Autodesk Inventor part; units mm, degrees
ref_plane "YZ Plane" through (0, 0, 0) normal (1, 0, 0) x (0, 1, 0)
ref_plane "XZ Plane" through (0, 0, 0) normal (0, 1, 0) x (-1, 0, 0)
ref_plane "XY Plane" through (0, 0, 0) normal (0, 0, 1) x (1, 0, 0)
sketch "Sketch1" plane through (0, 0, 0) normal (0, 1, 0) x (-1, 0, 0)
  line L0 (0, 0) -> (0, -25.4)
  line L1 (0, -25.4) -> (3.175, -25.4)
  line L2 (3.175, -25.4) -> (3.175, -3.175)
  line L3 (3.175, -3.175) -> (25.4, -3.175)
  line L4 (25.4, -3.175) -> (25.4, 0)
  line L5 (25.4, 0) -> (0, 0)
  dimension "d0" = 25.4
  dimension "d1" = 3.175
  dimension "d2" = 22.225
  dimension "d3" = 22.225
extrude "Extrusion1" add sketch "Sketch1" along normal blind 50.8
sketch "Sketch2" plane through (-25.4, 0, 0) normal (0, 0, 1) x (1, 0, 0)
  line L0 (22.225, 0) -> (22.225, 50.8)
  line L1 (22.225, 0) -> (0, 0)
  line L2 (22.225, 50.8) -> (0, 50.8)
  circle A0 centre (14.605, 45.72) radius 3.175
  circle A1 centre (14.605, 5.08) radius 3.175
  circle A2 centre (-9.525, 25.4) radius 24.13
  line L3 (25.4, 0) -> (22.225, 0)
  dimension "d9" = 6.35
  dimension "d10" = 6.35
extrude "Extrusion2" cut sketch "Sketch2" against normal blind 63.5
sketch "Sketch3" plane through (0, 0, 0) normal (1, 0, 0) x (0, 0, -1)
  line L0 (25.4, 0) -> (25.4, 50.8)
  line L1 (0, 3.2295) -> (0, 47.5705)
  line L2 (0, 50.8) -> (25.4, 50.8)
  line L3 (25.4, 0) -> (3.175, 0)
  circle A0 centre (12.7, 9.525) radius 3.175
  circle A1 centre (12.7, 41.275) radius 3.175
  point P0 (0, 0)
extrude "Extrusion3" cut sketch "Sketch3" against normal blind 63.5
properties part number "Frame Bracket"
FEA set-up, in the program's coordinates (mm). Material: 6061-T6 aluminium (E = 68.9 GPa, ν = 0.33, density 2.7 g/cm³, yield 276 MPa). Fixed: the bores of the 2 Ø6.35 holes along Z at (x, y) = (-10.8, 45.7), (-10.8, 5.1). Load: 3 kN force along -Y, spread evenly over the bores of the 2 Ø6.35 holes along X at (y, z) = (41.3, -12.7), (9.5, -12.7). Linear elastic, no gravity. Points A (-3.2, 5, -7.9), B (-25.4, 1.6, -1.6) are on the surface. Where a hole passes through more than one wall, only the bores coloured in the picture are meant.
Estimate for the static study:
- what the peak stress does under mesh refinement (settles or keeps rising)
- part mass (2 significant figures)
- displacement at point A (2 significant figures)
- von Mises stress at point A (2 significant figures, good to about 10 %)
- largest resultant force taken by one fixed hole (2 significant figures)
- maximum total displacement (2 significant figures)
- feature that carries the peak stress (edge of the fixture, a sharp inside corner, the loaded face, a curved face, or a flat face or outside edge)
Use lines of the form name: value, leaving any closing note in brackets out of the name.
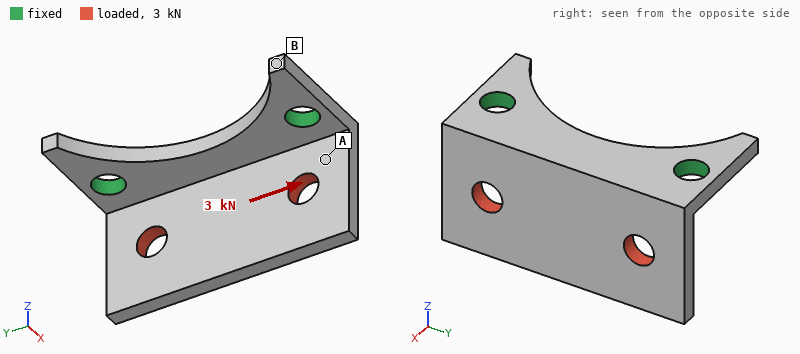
what the peak stress does under mesh refinement: keeps rising
part mass: 16 g
displacement at point A: 42 µm
von Mises stress at point A: 55 MPa
largest resultant force taken by one fixed hole: 1.8 kN
maximum total displacement: 100 µm
feature that carries the peak stress: edge of the fixture
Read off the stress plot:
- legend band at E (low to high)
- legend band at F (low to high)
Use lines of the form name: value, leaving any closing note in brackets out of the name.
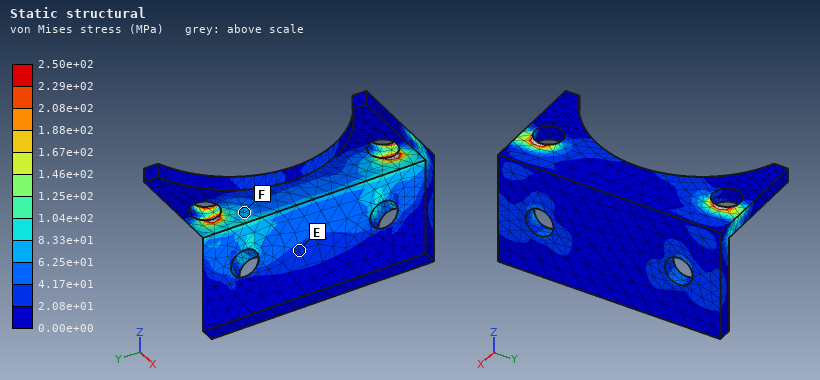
legend band at E: 2.08e+01 to 4.17e+01 MPa
legend band at F: 6.25e+01 to 8.33e+01 MPa
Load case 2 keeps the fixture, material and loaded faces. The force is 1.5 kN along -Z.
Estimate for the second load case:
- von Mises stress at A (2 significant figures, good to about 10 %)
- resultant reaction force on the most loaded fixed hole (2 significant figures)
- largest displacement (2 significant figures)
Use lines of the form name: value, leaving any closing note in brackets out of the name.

von Mises stress at A: 25 MPa
resultant reaction force on the most loaded fixed hole: 750 N
largest displacement: 0.15 mm
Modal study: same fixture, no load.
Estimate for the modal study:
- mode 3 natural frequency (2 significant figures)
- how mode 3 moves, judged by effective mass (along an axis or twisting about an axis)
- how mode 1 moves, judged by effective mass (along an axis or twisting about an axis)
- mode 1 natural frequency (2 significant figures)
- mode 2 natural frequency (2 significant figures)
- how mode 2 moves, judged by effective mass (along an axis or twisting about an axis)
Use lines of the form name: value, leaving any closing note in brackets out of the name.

mode 3 natural frequency: 10 kHz
how mode 3 moves, judged by effective mass: along Z
how mode 1 moves, judged by effective mass: along X
mode 1 natural frequency: 2900 Hz
mode 2 natural frequency: 5400 Hz
how mode 2 moves, judged by effective mass: twisting about Z
